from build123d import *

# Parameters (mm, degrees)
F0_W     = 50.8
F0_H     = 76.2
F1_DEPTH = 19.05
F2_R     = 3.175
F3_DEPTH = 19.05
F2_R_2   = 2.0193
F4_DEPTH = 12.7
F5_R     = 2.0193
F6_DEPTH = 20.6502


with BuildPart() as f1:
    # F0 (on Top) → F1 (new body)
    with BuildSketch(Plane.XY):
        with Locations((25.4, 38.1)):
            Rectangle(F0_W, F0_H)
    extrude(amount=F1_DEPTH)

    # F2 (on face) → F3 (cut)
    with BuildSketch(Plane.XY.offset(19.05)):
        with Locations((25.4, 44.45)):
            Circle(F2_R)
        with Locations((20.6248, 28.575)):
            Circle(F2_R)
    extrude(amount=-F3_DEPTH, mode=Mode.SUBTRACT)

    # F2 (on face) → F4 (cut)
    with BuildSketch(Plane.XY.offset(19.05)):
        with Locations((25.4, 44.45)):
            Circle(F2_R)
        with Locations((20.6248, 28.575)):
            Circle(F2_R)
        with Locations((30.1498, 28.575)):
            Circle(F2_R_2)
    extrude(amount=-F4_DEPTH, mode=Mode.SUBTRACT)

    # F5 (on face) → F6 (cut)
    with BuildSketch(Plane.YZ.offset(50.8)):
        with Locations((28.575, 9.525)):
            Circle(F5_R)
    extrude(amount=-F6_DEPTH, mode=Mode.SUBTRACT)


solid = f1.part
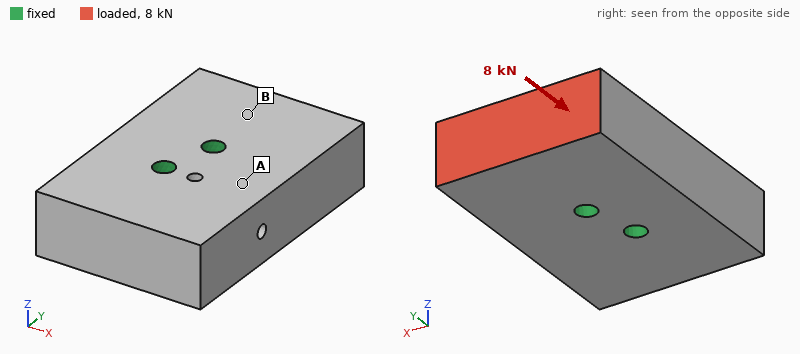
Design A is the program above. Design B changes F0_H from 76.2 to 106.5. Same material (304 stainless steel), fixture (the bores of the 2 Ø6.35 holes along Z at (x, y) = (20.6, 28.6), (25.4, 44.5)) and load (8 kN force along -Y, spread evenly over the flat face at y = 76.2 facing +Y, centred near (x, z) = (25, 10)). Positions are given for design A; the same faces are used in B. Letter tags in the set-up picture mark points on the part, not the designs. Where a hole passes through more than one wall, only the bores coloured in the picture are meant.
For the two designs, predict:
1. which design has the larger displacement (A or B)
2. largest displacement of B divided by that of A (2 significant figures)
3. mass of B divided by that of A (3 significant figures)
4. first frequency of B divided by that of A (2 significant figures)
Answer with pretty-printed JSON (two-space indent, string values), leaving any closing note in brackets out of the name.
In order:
{
  "which design has the larger displacement": "B",
  "largest displacement of B divided by that of A": "1.2",
  "mass of B divided by that of A": "1.41",
  "first frequency of B divided by that of A": "0.58"
}
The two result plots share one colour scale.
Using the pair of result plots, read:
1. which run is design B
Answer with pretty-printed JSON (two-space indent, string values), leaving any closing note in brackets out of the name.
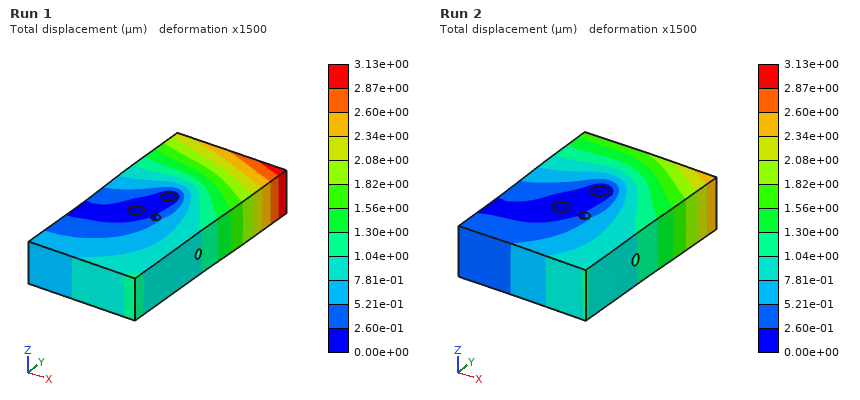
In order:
{
  "which run is design B": "Run 1"
}
